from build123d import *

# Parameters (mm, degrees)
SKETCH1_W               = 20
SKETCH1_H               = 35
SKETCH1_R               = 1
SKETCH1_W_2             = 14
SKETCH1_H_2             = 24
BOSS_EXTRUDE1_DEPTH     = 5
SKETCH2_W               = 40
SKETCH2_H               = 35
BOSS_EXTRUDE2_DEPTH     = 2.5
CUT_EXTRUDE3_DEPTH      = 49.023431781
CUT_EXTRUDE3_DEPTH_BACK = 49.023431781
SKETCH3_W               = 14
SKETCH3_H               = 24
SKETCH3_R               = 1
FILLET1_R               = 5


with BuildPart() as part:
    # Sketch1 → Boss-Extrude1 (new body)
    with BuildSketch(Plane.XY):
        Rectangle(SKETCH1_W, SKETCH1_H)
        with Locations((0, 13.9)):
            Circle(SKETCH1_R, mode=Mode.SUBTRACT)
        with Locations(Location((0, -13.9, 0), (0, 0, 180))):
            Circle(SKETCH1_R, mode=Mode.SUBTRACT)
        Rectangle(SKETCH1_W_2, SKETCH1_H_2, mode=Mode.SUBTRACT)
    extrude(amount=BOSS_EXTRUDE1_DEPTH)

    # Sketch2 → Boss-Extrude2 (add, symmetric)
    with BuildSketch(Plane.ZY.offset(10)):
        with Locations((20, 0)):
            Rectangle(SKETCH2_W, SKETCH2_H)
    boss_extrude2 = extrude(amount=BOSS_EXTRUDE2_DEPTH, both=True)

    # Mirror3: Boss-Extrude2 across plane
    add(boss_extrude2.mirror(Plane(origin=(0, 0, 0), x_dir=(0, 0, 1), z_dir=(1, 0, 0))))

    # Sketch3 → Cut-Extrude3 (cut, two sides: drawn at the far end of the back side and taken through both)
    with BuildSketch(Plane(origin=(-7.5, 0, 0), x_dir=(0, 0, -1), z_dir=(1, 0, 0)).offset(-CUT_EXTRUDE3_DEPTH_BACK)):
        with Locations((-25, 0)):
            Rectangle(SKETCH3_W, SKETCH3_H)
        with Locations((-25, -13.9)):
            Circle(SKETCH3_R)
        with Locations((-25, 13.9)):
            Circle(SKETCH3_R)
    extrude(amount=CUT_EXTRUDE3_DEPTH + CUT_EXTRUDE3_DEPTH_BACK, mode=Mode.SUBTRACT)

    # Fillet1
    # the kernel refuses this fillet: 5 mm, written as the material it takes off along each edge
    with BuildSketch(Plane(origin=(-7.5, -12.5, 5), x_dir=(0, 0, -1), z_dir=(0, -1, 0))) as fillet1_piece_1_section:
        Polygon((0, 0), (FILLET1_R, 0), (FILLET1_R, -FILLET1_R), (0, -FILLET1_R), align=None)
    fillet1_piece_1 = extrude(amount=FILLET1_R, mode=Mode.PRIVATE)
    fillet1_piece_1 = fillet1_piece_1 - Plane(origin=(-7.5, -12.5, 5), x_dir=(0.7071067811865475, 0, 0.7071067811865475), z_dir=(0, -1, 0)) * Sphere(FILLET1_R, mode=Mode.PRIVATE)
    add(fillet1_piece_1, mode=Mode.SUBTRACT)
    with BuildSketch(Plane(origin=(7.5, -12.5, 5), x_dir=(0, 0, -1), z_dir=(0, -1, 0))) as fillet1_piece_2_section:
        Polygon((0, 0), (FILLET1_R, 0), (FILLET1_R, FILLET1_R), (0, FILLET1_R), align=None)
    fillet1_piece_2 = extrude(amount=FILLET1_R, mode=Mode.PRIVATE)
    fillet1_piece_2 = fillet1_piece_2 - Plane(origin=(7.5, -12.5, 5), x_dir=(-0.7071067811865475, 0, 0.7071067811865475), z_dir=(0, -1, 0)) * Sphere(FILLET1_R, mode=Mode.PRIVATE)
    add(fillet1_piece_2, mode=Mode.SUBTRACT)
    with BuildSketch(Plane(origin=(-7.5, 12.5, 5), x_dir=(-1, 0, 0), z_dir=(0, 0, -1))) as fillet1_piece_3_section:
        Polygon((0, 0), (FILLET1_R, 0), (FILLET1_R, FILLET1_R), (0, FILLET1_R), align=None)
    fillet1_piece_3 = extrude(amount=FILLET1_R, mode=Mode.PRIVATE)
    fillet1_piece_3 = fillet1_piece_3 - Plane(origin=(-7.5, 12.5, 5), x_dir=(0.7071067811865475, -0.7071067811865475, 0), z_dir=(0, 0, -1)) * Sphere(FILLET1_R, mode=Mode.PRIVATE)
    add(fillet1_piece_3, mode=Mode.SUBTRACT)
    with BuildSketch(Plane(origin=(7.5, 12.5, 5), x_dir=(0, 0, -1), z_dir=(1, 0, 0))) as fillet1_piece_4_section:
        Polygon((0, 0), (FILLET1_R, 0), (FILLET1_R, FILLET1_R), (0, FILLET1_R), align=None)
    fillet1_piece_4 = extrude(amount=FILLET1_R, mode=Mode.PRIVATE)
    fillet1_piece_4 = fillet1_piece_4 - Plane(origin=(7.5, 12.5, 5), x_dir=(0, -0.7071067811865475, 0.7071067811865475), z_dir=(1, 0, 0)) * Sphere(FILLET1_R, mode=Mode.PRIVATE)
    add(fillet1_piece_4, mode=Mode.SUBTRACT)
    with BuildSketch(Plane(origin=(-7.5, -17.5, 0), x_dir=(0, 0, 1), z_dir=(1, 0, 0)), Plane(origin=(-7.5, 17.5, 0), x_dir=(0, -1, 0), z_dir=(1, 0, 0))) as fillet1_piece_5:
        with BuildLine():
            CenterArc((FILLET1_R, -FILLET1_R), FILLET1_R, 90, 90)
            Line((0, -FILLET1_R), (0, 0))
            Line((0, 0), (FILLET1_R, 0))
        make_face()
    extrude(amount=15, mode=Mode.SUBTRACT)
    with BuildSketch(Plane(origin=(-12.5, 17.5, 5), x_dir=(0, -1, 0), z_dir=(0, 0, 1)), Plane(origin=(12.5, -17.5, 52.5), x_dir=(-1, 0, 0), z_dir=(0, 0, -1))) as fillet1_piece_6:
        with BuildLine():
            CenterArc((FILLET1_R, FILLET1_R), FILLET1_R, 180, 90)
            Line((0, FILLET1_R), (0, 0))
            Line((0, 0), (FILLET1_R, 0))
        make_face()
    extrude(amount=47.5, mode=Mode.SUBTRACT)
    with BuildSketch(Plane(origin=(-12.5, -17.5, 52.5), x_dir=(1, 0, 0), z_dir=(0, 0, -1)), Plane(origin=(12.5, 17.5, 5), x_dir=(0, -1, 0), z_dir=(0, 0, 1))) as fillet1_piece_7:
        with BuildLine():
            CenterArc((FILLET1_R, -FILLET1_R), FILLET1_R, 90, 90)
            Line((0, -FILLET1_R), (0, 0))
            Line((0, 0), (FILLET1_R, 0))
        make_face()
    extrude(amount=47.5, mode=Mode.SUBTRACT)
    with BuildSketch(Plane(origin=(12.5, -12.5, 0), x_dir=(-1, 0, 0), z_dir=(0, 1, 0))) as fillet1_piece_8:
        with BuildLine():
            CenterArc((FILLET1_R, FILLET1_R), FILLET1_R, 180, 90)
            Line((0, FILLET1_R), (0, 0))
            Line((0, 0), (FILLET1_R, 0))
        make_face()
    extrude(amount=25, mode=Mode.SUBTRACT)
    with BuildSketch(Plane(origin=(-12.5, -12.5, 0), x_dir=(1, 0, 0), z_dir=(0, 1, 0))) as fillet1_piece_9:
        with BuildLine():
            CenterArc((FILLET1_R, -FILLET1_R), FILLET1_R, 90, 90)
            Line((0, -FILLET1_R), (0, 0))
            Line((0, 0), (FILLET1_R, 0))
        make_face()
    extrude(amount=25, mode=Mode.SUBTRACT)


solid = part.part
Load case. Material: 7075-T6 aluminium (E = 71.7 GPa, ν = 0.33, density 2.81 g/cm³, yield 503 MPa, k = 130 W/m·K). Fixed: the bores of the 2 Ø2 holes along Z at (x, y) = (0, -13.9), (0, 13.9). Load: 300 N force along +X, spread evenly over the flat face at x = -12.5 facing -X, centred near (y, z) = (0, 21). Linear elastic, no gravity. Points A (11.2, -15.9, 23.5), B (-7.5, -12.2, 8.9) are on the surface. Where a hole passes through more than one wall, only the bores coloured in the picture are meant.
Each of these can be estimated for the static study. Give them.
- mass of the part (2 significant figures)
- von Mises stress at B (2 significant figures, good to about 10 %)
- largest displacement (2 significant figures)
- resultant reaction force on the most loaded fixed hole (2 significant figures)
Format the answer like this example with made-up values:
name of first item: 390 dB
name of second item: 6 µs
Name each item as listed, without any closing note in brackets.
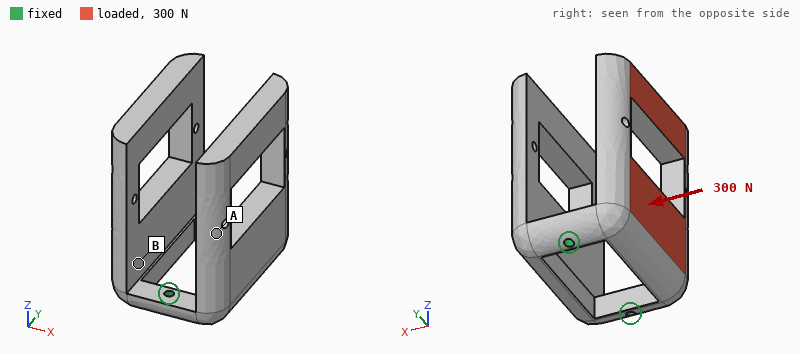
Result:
mass of the part: 28 g
von Mises stress at B: 41 MPa
largest displacement: 0.52 mm
resultant reaction force on the most loaded fixed hole: 190 N
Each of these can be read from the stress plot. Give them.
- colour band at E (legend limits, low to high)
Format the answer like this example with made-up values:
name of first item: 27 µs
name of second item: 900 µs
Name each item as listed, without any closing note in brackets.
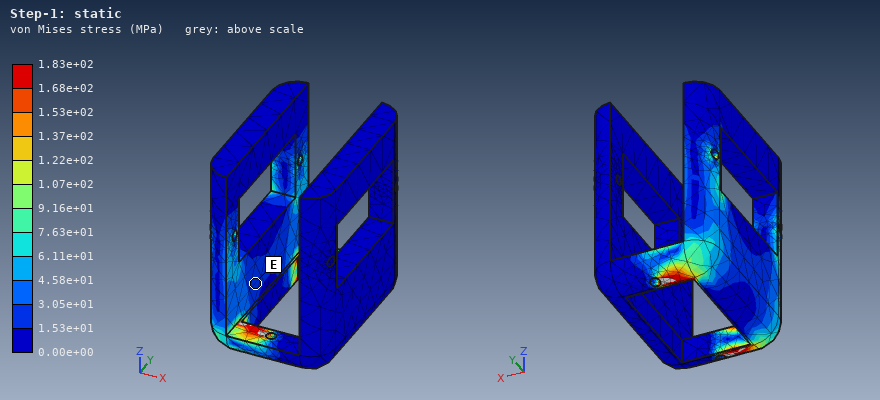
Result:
colour band at E: 1.53e+01 to 3.05e+01 MPa
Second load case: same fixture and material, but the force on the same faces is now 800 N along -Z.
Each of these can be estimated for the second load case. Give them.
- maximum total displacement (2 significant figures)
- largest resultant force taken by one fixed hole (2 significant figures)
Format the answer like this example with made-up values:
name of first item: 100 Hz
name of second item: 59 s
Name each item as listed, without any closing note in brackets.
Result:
maximum total displacement: 0.48 mm
largest resultant force taken by one fixed hole: 410 N
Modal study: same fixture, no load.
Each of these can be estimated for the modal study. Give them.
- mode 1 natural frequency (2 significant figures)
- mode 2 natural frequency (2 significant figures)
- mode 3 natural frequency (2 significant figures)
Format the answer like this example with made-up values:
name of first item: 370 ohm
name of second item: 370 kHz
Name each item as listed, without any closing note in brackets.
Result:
mode 1 natural frequency: 1300 Hz
mode 2 natural frequency: 1400 Hz
mode 3 natural frequency: 3800 Hz
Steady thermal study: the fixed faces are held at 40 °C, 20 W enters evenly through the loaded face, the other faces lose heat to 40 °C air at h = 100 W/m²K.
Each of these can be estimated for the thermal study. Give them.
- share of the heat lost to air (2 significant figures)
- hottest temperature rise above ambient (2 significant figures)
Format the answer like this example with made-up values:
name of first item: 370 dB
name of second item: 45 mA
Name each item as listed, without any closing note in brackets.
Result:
share of the heat lost to air: 38 %
hottest temperature rise above ambient: 44 K
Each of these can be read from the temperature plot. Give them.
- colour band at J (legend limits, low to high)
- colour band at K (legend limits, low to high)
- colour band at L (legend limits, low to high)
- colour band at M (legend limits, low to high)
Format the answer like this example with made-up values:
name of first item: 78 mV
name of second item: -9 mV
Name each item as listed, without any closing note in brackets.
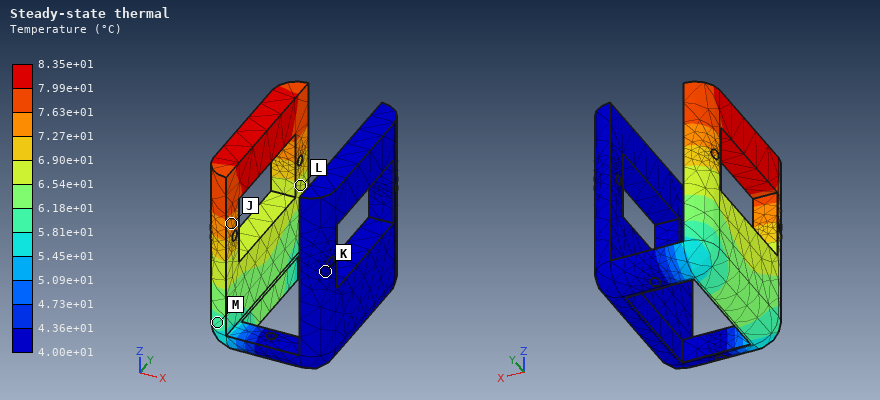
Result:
colour band at J: 7.27e+01 to 7.63e+01 °C
colour band at K: 4.00e+01 to 4.36e+01 °C
colour band at L: 6.54e+01 to 6.90e+01 °C
colour band at M: 5.81e+01 to 6.18e+01 °C
